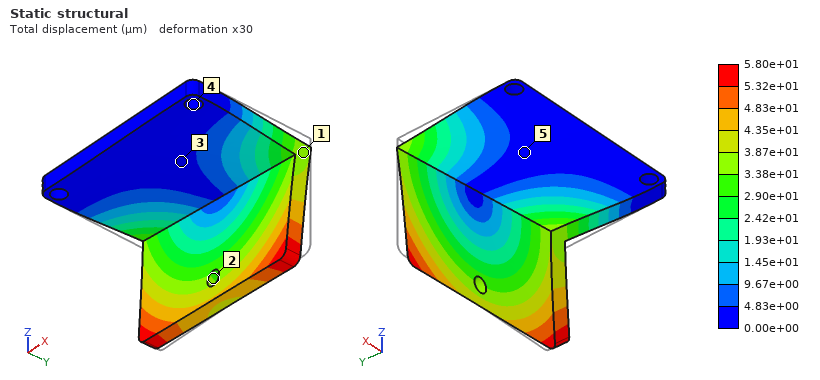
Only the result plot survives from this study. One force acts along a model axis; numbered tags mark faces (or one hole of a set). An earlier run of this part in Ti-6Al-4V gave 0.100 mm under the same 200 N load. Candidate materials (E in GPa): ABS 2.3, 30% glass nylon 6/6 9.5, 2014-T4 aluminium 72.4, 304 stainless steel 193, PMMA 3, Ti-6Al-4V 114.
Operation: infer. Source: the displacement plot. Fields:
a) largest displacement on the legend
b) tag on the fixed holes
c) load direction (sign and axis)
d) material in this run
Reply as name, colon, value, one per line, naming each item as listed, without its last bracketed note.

largest displacement on the legend: 5.80e+01 µm
tag on the fixed holes: 4
load direction: -X
material in this run: 304 stainless steel
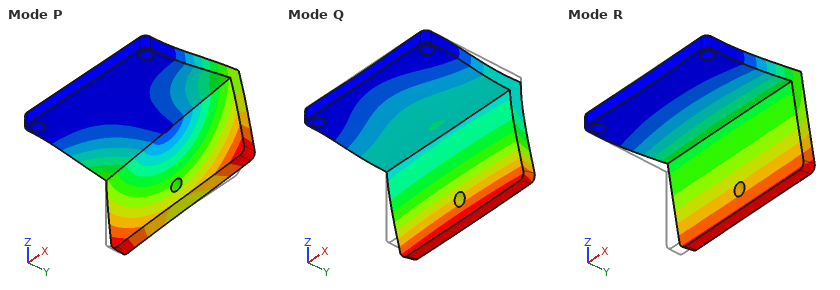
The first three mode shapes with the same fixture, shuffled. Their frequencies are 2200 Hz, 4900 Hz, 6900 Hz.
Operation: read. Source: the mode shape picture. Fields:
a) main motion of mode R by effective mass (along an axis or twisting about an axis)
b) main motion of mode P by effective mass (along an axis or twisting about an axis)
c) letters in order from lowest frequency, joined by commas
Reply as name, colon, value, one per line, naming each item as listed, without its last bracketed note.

main motion of mode R by effective mass: along Z
main motion of mode P by effective mass: along X
letters in order from lowest frequency, joined by commas: R, P, Q
